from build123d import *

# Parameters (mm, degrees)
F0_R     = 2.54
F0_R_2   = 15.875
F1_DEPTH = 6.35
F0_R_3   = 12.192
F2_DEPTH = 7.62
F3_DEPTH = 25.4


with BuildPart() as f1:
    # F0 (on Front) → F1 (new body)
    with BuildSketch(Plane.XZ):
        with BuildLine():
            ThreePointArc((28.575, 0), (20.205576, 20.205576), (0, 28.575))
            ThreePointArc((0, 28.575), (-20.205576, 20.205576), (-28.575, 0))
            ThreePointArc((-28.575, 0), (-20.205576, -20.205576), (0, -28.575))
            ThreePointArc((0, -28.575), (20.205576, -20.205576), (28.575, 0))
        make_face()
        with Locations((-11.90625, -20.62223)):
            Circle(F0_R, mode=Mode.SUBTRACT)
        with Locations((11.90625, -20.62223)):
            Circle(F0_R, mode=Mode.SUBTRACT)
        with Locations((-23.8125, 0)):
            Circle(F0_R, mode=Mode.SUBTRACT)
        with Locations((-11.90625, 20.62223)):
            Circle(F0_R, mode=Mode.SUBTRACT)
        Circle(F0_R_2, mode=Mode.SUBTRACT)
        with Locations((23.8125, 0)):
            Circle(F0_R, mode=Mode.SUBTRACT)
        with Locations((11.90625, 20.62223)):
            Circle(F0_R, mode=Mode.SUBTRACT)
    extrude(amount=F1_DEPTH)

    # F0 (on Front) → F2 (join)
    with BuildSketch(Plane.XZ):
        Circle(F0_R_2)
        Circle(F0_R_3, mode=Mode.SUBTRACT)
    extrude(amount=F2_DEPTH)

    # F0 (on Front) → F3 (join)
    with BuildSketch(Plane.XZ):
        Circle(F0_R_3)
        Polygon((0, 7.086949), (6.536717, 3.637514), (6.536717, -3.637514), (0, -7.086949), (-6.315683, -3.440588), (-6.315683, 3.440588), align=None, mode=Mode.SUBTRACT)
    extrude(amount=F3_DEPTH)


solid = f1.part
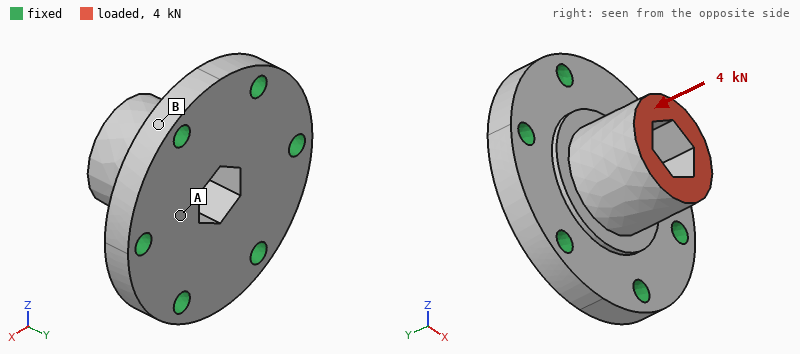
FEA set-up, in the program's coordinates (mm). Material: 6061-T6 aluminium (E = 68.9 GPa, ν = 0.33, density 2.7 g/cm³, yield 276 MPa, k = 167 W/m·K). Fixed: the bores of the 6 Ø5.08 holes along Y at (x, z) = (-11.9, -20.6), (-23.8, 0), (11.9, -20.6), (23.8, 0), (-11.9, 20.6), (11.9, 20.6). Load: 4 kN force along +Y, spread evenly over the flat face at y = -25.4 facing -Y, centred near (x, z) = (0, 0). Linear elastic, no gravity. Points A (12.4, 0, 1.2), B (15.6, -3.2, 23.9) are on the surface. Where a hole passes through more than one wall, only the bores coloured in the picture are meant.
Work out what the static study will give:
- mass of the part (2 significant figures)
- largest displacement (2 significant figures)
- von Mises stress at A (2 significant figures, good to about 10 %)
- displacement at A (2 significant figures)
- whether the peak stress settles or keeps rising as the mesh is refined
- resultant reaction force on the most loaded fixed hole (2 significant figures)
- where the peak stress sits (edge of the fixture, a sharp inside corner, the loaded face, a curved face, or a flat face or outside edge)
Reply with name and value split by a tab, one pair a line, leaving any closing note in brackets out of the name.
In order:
mass of the part	58 g
largest displacement	12 µm
von Mises stress at A	14 MPa
displacement at A	7.8 µm
whether the peak stress settles or keeps rising as the mesh is refined	keeps rising
resultant reaction force on the most loaded fixed hole	760 N
where the peak stress sits	edge of the fixture
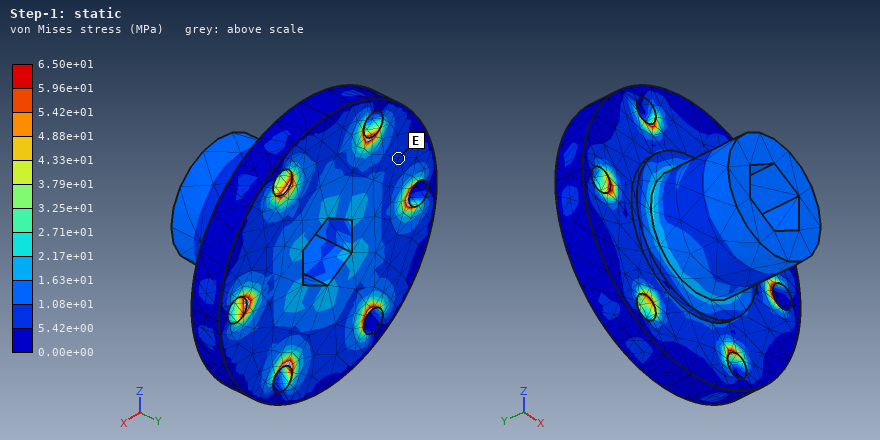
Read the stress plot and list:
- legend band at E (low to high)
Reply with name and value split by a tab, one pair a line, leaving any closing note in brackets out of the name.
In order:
legend band at E	5.42e+00 to 1.08e+01 MPa
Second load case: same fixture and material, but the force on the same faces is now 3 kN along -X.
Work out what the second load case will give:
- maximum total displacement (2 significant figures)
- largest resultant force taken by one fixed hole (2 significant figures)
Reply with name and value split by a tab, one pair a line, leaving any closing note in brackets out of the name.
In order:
maximum total displacement	40 µm
largest resultant force taken by one fixed hole	1.4 kN
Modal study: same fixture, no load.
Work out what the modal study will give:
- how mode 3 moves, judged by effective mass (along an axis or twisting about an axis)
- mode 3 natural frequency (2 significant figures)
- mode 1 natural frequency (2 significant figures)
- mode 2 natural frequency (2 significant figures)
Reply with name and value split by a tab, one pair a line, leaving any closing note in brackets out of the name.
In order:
how mode 3 moves, judged by effective mass	along Y
mode 3 natural frequency	19 kHz
mode 1 natural frequency	18 kHz
mode 2 natural frequency	18 kHz
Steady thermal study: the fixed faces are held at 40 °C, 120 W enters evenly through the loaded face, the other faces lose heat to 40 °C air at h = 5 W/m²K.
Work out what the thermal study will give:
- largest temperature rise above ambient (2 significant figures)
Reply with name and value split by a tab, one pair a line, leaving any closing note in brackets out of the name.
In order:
largest temperature rise above ambient	57 K
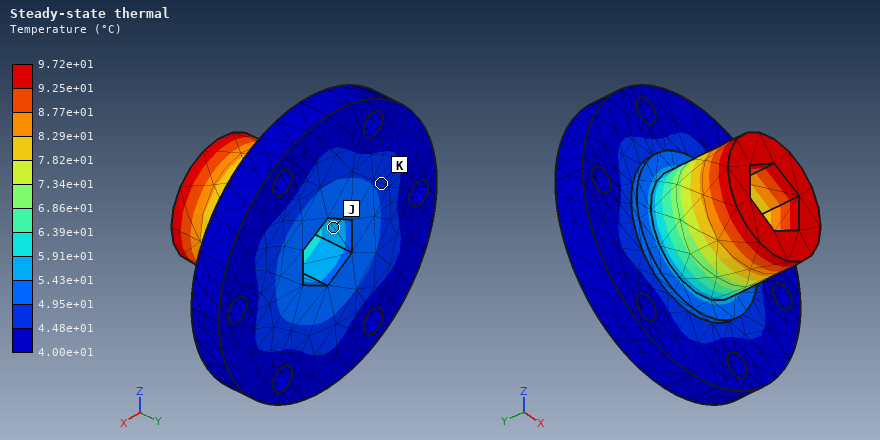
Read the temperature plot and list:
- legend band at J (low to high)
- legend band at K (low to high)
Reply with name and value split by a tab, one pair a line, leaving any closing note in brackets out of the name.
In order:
legend band at J	5.43e+01 to 5.91e+01 °C
legend band at K	4.48e+01 to 4.95e+01 °C
